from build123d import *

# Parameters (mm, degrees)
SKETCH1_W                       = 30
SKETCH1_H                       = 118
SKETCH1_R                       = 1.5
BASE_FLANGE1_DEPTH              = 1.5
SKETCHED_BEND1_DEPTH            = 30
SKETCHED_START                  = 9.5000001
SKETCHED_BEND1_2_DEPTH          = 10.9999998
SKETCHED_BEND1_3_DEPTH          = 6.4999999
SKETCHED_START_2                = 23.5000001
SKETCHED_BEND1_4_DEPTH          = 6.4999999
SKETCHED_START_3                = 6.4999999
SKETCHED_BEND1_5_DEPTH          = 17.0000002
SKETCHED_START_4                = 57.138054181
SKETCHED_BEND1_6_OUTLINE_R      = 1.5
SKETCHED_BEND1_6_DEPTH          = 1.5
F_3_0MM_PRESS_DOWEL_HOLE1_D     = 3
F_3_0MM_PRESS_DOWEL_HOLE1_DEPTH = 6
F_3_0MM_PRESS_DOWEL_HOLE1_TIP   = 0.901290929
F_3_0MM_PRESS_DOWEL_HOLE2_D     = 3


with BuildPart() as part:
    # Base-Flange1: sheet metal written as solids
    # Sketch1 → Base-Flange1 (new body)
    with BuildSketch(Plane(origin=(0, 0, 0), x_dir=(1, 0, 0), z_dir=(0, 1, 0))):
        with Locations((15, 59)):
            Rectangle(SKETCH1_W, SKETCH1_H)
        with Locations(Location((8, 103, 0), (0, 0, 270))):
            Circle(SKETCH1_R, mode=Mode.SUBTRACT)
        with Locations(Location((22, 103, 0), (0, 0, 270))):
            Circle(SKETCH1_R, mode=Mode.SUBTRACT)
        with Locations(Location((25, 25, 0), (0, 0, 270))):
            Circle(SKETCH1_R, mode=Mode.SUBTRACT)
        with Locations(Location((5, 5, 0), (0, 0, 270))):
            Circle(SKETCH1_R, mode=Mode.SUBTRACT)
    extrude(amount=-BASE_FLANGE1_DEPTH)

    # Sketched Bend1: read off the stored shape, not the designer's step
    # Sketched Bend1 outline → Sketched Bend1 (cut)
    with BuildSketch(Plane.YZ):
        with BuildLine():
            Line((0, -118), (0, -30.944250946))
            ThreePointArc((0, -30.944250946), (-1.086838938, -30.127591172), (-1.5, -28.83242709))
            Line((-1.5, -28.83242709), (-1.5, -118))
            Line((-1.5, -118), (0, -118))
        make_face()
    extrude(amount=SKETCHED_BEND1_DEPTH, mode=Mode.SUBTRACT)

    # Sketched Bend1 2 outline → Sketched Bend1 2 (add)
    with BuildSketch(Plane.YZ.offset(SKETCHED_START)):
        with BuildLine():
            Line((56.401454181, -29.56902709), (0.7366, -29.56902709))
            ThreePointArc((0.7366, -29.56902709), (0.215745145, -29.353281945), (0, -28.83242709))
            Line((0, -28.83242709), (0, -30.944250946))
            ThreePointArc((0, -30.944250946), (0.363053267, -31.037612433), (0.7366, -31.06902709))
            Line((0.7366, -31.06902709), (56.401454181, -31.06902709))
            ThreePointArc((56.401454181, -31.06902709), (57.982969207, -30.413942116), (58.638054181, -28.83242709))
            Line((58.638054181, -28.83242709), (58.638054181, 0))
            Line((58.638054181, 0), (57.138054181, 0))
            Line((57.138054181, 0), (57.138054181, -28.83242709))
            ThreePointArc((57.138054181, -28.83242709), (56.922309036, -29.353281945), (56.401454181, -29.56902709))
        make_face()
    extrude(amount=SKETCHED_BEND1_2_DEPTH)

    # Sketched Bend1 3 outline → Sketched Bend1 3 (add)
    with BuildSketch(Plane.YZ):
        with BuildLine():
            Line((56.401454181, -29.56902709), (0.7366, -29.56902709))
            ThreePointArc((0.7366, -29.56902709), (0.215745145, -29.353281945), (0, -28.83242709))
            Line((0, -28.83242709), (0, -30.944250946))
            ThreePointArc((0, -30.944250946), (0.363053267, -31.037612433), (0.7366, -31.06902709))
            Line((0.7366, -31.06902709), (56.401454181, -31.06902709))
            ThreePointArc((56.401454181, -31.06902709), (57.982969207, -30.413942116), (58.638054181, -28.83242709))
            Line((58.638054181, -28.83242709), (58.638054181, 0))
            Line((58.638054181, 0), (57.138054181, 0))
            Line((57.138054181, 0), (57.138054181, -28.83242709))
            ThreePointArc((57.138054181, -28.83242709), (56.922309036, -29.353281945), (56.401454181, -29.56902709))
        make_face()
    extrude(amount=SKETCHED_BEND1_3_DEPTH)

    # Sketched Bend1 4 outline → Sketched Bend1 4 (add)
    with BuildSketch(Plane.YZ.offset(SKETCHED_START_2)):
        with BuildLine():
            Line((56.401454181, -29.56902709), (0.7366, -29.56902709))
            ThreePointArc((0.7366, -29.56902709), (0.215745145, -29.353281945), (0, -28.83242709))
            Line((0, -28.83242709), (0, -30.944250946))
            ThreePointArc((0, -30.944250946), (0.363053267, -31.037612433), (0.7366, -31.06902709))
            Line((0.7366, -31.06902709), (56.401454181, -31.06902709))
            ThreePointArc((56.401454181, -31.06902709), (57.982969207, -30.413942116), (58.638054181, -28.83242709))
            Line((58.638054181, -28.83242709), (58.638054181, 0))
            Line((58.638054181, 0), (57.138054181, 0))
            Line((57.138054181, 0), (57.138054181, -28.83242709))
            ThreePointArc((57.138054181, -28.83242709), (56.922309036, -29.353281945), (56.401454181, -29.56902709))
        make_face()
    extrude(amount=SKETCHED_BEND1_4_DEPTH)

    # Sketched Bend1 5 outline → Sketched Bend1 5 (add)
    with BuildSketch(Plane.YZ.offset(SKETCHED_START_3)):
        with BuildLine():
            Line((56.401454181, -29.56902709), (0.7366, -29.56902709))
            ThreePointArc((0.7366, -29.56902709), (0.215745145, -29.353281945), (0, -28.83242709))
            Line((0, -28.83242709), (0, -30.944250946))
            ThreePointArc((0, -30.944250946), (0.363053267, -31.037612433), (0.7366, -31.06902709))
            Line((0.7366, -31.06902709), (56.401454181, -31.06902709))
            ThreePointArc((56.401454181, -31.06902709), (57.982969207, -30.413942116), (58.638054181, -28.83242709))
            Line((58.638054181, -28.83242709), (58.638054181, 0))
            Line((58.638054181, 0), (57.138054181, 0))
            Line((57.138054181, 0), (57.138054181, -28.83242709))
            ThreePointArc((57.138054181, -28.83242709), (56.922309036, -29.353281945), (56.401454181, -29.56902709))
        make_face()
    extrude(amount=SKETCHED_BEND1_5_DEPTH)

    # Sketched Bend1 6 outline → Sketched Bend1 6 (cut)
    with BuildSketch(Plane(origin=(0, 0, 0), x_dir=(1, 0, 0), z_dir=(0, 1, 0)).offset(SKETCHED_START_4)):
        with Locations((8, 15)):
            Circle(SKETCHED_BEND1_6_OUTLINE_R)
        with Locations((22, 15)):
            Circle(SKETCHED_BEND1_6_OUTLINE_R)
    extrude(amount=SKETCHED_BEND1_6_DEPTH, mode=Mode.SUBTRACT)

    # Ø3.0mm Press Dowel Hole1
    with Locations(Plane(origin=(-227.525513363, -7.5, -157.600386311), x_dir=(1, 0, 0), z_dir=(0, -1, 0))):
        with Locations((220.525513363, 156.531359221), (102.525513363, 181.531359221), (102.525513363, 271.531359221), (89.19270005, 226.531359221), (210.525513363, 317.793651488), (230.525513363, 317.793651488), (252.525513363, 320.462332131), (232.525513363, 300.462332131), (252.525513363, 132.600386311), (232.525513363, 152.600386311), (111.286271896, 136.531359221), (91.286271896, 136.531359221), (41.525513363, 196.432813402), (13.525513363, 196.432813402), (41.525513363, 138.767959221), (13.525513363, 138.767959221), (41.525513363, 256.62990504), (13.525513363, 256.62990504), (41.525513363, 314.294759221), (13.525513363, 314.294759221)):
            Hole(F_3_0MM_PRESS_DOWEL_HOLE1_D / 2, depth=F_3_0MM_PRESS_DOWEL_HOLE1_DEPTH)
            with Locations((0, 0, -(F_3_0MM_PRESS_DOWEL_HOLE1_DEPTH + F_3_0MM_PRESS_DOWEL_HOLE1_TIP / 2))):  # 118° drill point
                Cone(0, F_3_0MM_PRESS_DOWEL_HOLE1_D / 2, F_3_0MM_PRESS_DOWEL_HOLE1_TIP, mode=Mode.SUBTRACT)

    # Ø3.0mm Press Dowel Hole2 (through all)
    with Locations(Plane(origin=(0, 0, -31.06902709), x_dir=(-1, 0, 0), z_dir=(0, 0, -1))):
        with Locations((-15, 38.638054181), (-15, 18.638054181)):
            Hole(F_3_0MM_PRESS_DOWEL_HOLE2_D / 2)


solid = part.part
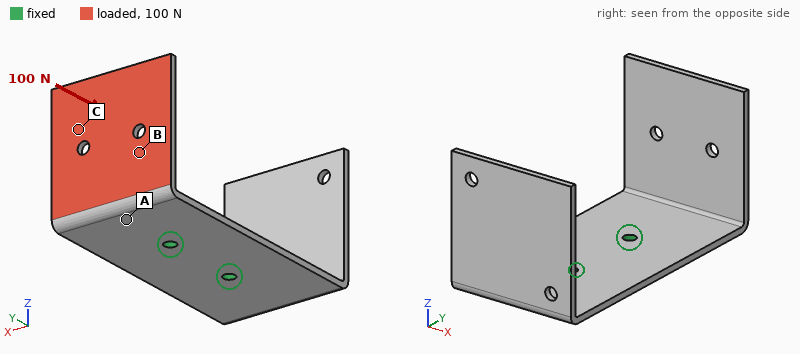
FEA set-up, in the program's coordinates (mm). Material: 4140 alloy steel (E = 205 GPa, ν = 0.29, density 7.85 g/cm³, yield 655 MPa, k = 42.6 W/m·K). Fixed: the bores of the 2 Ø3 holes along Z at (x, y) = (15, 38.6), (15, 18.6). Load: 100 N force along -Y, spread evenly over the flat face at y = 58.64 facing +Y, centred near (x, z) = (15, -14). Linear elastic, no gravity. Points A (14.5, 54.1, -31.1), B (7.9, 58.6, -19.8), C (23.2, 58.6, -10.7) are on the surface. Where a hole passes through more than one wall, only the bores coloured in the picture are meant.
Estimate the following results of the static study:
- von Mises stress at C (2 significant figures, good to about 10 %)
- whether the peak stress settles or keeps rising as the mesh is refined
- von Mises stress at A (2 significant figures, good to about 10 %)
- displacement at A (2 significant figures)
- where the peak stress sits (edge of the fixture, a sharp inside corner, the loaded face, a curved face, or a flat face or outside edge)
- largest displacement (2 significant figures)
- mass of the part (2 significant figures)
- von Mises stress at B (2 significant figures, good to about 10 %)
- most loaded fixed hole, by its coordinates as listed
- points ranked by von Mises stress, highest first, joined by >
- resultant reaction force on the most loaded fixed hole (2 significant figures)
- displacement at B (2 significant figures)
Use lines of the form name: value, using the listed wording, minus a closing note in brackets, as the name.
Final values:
von Mises stress at C: 16 MPa
whether the peak stress settles or keeps rising as the mesh is refined: keeps rising
von Mises stress at A: 130 MPa
displacement at A: 0.12 mm
where the peak stress sits: edge of the fixture
largest displacement: 0.75 mm
mass of the part: 41 g
von Mises stress at B: 53 MPa
most loaded fixed hole, by its coordinates as listed: (15, 38.6)
points ranked by von Mises stress, highest first, joined by >: A > B > C
resultant reaction force on the most loaded fixed hole: 80 N
displacement at B: 0.29 mm
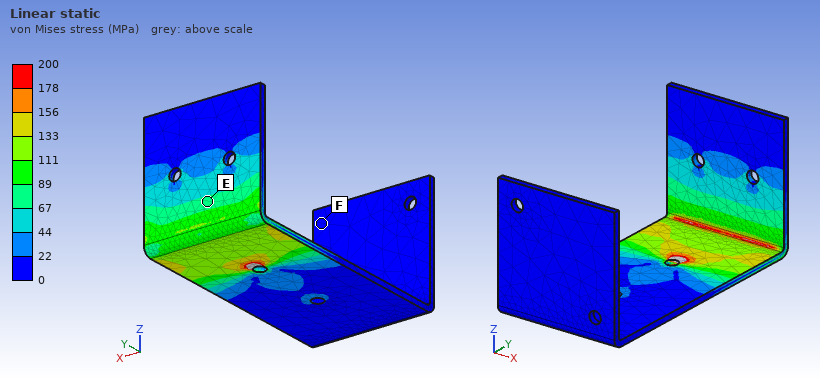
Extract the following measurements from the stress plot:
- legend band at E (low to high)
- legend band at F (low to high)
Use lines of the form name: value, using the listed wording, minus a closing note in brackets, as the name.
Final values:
legend band at E: 67 to 89 MPa
legend band at F: 0 to 22 MPa
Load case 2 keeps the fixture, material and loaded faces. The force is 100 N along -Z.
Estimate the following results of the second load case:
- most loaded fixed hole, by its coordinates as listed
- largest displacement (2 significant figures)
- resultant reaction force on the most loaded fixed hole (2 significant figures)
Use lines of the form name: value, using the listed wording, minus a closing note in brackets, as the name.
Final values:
most loaded fixed hole, by its coordinates as listed: (15, 38.6)
largest displacement: 0.42 mm
resultant reaction force on the most loaded fixed hole: 130 N
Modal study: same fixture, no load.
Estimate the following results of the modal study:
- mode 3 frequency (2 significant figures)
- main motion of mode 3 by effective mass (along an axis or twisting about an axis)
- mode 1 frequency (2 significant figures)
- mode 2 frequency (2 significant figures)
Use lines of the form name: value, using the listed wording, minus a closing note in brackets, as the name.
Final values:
mode 3 frequency: 940 Hz
main motion of mode 3 by effective mass: along X
mode 1 frequency: 640 Hz
mode 2 frequency: 660 Hz
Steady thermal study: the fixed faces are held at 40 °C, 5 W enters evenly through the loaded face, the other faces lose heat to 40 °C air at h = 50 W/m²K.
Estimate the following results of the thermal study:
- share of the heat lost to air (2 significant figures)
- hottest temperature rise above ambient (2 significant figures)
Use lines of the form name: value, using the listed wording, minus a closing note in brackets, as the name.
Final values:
share of the heat lost to air: 66 %
hottest temperature rise above ambient: 48 K
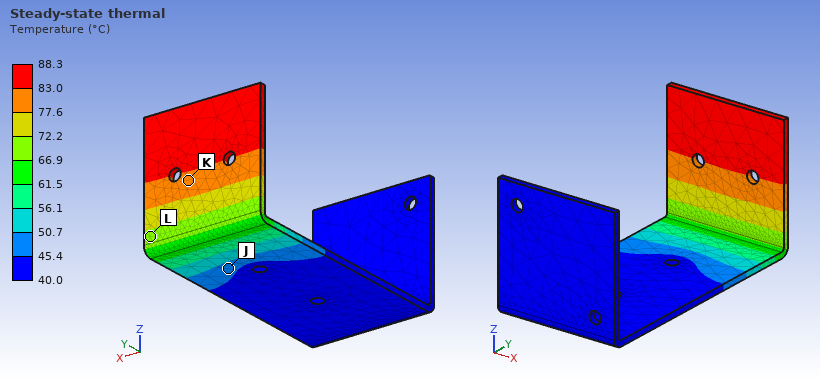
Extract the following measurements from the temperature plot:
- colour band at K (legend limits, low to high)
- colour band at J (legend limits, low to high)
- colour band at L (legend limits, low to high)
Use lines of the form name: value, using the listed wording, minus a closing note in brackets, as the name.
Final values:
colour band at K: 77.6 to 83.0 °C
colour band at J: 45.4 to 50.7 °C
colour band at L: 66.9 to 72.2 °C
